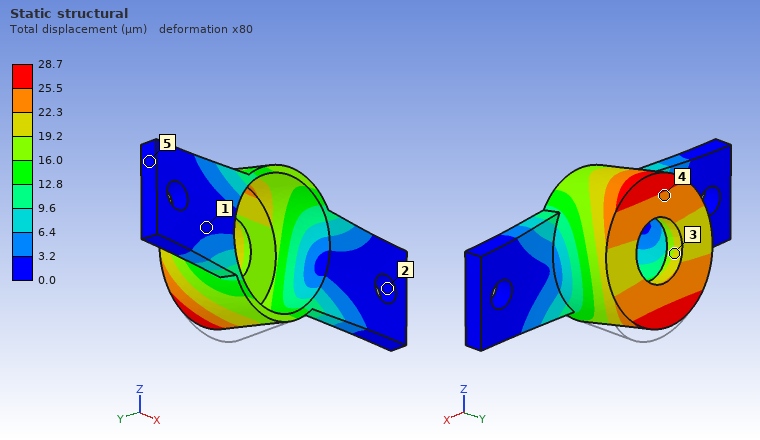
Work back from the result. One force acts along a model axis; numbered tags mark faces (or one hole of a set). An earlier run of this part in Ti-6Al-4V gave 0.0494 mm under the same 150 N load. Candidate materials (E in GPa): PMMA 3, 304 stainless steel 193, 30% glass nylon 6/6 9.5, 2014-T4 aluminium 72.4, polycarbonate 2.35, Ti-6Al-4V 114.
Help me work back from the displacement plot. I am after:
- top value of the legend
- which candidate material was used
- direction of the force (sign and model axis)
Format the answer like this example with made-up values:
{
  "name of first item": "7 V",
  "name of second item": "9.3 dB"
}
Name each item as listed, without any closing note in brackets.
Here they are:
{
  "top value of the legend": "28.7 µm",
  "which candidate material was used": "304 stainless steel",
  "direction of the force": "+Z"
}
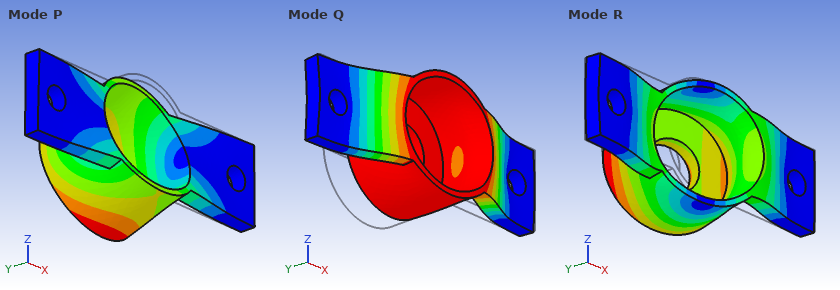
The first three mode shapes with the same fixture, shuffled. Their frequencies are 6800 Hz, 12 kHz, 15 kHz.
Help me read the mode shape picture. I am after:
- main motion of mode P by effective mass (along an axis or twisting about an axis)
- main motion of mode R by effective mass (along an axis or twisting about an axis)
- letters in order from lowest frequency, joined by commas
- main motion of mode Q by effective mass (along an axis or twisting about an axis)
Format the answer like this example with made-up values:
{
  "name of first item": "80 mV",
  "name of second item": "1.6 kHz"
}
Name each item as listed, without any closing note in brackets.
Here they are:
{
  "main motion of mode P by effective mass": "along Z",
  "main motion of mode R by effective mass": "along X",
  "letters in order from lowest frequency, joined by commas": "P, Q, R",
  "main motion of mode Q by effective mass": "along Y"
}
